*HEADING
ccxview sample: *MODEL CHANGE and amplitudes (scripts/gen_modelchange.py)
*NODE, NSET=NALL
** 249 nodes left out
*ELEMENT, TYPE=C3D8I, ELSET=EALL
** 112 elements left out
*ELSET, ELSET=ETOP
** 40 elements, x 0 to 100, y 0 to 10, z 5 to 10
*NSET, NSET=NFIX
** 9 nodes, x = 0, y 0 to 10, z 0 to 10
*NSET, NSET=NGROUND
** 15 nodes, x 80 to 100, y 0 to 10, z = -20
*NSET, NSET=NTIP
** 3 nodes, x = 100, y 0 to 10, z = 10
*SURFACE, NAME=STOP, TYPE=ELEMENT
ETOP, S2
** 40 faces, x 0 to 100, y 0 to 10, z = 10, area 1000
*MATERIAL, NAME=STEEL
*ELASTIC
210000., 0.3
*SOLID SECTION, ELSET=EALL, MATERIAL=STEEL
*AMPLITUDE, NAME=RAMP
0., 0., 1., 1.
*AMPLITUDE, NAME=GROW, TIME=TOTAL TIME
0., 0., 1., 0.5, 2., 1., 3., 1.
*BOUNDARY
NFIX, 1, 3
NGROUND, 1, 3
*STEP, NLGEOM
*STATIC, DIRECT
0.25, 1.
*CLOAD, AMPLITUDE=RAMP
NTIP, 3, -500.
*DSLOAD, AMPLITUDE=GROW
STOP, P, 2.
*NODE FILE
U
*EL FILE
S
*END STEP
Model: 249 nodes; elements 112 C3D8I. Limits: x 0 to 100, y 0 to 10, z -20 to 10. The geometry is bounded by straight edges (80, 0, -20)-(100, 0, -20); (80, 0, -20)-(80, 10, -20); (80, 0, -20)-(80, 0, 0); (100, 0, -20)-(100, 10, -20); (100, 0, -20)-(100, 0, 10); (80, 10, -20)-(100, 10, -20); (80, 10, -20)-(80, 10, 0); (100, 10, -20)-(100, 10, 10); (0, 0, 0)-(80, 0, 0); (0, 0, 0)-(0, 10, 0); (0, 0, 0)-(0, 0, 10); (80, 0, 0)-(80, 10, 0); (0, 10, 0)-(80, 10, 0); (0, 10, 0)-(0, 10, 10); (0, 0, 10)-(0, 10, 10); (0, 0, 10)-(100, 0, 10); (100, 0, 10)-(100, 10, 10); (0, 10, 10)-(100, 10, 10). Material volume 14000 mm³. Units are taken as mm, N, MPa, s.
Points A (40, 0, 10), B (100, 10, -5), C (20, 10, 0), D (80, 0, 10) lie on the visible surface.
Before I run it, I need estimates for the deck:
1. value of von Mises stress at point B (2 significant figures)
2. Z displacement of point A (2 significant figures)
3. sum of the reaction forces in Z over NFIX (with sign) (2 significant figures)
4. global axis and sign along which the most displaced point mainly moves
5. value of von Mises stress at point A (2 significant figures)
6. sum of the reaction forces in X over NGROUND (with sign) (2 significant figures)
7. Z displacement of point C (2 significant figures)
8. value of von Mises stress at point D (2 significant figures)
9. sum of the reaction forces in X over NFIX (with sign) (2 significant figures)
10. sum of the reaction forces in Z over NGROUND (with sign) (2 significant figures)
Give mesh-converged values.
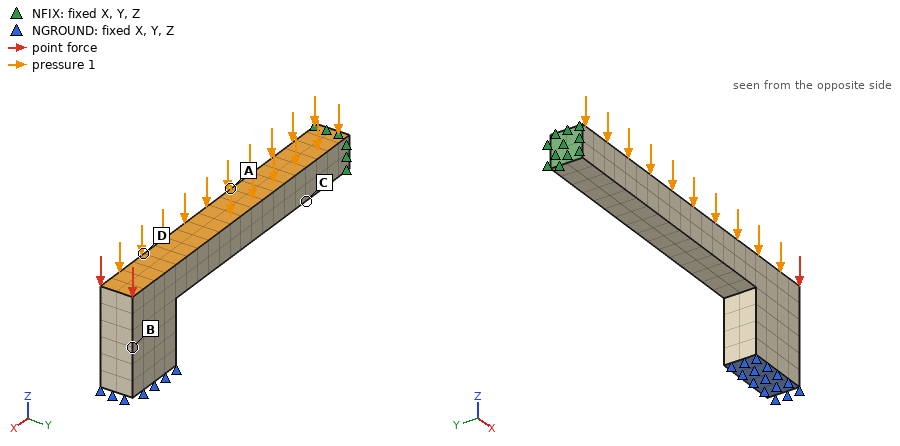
21 MPa
-0.0083 mm
420 N
-Z
16 MPa
120 N
-0.0046 mm
25 MPa
-120 N
2100 N
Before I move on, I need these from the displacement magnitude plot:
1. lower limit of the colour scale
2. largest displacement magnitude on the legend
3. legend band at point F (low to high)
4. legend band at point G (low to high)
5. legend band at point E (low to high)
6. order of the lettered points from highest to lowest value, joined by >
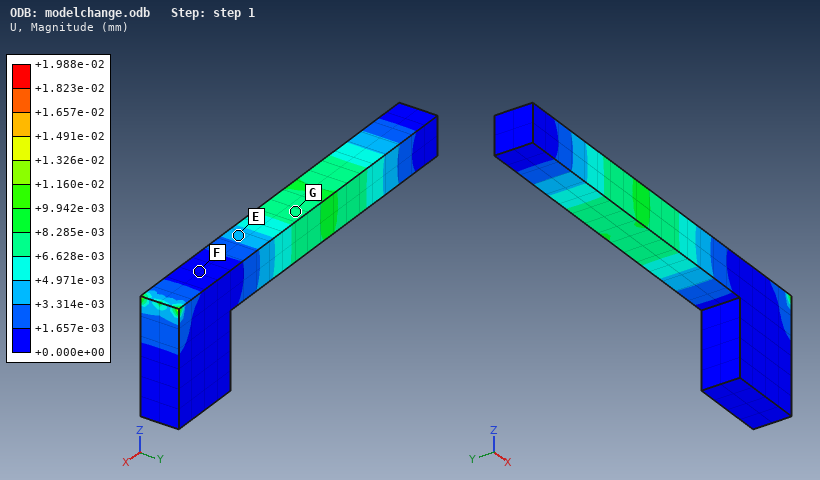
+0.000e+00 mm
+1.988e-02 mm
+0.000e+00 to +1.657e-03 mm
+6.628e-03 to +8.285e-03 mm
+3.314e-03 to +4.971e-03 mm
G > E > F
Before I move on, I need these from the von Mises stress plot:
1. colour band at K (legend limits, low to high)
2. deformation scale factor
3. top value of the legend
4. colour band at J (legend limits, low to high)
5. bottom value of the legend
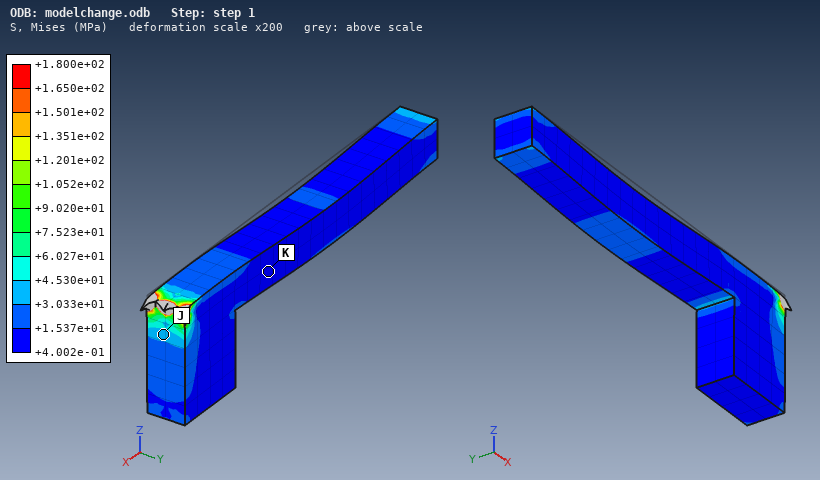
+4.002e-01 to +1.537e+01 MPa
200
+1.800e+02 MPa
+3.033e+01 to +4.530e+01 MPa
+4.002e-01 MPa
